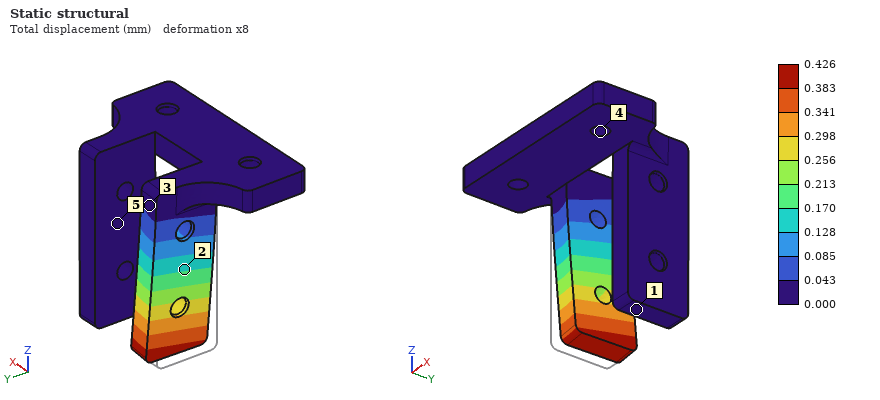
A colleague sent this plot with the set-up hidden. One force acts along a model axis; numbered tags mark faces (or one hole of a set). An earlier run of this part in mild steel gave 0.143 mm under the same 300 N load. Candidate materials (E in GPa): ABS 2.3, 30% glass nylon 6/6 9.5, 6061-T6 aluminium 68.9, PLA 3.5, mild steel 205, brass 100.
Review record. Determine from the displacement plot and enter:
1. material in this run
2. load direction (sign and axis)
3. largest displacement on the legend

6061-T6 aluminium
+X
0.426 mm
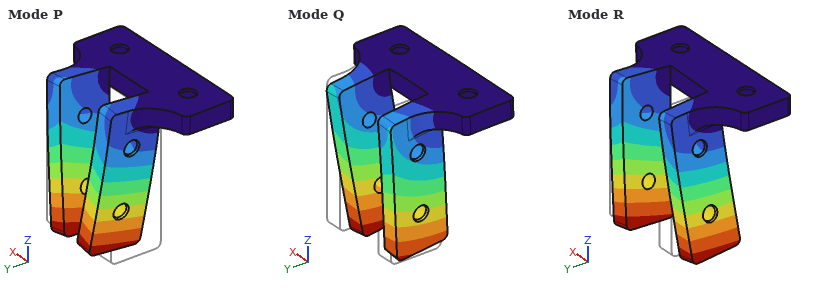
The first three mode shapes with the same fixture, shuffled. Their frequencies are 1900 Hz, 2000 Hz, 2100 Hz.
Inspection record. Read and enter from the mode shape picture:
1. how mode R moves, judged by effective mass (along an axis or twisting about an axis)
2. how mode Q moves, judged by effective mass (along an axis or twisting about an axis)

along X
along Y
